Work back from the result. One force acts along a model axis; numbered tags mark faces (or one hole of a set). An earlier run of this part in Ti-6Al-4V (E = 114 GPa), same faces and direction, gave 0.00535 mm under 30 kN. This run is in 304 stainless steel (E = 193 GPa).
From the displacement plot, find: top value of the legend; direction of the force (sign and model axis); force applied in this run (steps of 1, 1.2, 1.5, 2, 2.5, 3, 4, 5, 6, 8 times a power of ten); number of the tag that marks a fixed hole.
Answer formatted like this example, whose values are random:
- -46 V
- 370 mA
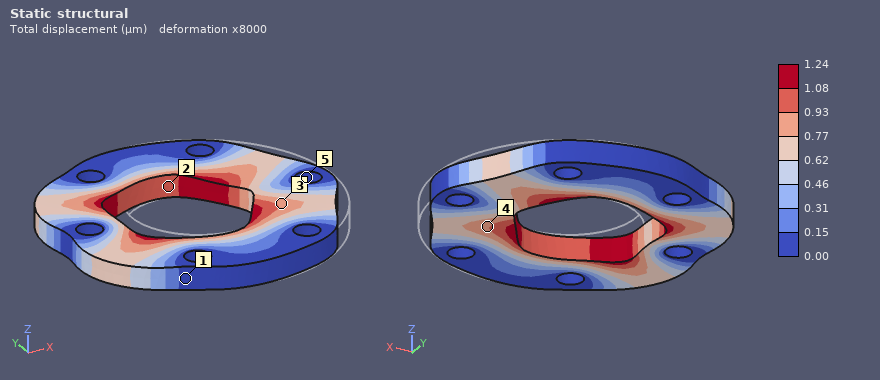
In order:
- 1.24 µm
- -X
- 12 kN
- 5
